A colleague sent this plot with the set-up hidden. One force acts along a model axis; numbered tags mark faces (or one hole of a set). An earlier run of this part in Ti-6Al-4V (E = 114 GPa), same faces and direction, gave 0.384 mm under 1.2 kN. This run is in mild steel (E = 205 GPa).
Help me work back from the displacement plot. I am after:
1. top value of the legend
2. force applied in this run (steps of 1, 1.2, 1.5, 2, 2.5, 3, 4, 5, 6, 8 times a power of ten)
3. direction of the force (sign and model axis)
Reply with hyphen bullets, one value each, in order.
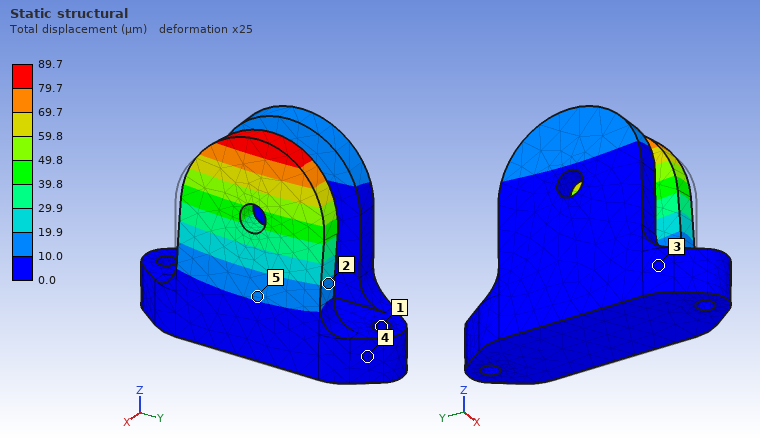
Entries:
- 89.7 µm
- 500 N
- -X
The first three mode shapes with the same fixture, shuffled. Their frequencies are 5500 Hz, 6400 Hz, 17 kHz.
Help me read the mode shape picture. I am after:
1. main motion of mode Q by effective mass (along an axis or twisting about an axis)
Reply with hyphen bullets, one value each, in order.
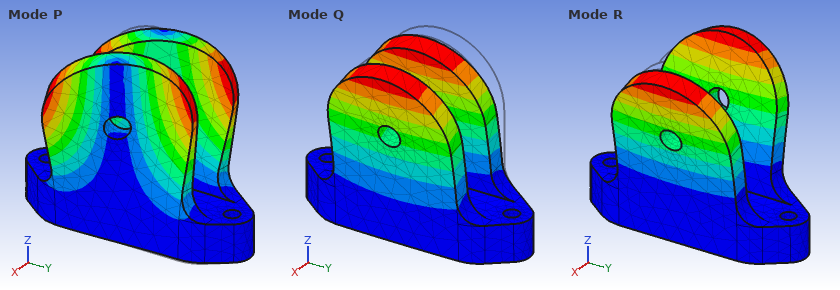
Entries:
- along X
